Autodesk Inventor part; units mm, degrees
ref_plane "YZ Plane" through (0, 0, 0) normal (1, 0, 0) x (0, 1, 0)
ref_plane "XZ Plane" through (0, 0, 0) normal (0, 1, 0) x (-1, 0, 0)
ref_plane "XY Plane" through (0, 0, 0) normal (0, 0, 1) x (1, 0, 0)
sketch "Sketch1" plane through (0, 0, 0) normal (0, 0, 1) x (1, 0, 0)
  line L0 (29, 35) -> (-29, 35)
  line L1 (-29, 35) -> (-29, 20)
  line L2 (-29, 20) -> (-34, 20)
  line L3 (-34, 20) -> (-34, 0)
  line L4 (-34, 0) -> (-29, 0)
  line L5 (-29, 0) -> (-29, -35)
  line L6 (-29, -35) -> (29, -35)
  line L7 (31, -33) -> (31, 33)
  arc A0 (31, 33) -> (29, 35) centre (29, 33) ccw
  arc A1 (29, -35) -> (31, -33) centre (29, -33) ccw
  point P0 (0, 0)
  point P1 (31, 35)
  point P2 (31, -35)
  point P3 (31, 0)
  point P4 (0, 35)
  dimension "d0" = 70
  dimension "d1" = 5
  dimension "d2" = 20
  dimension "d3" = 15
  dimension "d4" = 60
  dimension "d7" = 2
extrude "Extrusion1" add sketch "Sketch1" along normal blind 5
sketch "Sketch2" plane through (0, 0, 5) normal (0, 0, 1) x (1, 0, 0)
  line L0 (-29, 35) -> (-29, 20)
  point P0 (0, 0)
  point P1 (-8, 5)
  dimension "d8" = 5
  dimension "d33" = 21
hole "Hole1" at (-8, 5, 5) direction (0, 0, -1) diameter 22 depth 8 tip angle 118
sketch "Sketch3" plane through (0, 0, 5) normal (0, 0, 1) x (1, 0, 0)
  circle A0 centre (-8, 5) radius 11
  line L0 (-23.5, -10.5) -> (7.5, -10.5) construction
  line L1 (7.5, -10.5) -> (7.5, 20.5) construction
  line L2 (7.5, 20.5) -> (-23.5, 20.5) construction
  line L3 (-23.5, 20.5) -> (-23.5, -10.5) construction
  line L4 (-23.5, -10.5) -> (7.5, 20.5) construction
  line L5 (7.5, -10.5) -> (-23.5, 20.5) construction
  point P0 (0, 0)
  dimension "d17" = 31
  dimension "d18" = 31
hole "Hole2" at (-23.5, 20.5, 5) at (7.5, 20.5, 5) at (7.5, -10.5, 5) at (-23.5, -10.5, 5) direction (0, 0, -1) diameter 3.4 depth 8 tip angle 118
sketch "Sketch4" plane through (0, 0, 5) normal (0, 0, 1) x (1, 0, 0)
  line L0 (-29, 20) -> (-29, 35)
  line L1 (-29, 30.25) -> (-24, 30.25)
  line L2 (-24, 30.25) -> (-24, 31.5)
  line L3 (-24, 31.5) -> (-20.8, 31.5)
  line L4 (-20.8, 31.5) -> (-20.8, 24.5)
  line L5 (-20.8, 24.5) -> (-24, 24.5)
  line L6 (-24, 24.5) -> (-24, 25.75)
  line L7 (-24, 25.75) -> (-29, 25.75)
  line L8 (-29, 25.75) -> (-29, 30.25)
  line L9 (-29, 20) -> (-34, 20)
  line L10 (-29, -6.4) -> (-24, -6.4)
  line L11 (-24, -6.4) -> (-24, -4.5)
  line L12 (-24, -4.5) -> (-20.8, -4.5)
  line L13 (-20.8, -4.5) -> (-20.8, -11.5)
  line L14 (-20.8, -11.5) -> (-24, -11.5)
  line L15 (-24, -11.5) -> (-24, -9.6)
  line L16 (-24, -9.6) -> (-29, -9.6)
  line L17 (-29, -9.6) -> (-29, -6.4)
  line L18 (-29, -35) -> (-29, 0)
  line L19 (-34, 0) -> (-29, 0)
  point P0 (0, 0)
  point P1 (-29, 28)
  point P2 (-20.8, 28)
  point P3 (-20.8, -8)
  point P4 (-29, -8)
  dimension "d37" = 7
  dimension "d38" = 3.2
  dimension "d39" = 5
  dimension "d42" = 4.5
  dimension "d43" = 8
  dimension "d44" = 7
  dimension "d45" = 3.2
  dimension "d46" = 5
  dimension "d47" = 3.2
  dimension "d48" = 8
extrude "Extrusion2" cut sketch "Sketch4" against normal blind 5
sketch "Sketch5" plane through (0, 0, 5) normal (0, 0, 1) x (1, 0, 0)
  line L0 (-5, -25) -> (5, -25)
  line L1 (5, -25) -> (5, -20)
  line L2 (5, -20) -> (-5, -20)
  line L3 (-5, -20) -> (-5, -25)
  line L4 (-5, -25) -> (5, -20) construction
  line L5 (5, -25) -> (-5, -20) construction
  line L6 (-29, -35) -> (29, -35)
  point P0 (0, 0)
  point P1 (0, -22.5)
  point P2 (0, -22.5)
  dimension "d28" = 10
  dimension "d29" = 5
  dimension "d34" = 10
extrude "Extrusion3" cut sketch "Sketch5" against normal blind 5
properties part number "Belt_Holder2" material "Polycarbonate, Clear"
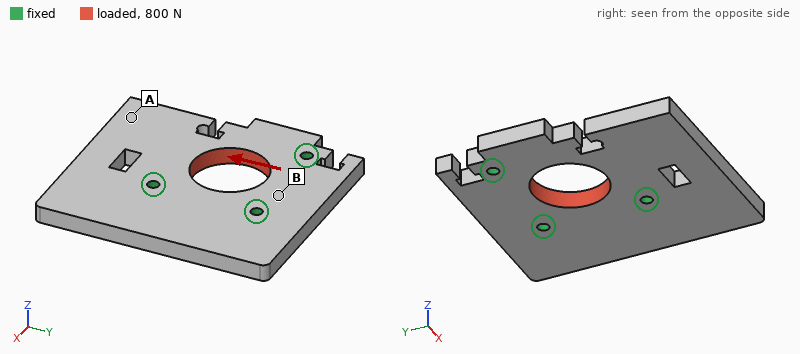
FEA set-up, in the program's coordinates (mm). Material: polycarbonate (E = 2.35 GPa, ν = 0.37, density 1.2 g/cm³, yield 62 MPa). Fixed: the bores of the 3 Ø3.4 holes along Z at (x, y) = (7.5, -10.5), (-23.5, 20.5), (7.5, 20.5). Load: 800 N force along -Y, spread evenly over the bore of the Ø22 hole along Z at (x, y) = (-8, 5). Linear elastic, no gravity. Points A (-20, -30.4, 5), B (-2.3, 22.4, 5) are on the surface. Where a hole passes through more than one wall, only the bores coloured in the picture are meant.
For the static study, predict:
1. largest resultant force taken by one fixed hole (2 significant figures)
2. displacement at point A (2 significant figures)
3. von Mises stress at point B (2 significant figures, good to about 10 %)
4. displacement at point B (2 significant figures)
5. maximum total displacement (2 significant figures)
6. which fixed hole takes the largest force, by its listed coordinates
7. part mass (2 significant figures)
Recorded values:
350 N
75 µm
2.0 MPa
21 µm
95 µm
(-23.5, 20.5)
23 g
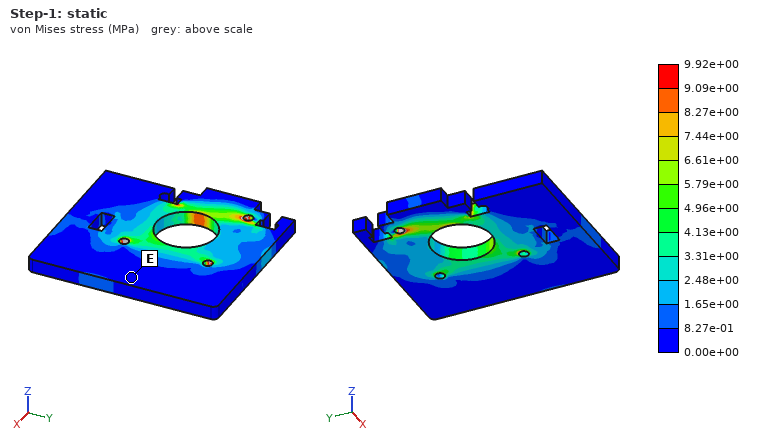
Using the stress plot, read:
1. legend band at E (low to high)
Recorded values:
0.00e+00 to 8.27e-01 MPa
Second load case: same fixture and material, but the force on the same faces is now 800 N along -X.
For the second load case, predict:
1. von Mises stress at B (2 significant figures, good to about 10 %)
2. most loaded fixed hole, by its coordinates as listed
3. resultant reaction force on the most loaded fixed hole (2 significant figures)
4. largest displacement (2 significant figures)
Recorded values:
2.0 MPa
(7.5, -10.5)
380 N
93 µm
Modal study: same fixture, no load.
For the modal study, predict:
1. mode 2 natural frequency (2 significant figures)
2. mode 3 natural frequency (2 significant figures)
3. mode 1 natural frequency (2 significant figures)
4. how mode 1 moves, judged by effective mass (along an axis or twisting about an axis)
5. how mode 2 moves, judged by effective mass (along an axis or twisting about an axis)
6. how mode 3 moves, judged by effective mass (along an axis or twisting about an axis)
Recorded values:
1400 Hz
1800 Hz
780 Hz
along Z
along Z
along Z
